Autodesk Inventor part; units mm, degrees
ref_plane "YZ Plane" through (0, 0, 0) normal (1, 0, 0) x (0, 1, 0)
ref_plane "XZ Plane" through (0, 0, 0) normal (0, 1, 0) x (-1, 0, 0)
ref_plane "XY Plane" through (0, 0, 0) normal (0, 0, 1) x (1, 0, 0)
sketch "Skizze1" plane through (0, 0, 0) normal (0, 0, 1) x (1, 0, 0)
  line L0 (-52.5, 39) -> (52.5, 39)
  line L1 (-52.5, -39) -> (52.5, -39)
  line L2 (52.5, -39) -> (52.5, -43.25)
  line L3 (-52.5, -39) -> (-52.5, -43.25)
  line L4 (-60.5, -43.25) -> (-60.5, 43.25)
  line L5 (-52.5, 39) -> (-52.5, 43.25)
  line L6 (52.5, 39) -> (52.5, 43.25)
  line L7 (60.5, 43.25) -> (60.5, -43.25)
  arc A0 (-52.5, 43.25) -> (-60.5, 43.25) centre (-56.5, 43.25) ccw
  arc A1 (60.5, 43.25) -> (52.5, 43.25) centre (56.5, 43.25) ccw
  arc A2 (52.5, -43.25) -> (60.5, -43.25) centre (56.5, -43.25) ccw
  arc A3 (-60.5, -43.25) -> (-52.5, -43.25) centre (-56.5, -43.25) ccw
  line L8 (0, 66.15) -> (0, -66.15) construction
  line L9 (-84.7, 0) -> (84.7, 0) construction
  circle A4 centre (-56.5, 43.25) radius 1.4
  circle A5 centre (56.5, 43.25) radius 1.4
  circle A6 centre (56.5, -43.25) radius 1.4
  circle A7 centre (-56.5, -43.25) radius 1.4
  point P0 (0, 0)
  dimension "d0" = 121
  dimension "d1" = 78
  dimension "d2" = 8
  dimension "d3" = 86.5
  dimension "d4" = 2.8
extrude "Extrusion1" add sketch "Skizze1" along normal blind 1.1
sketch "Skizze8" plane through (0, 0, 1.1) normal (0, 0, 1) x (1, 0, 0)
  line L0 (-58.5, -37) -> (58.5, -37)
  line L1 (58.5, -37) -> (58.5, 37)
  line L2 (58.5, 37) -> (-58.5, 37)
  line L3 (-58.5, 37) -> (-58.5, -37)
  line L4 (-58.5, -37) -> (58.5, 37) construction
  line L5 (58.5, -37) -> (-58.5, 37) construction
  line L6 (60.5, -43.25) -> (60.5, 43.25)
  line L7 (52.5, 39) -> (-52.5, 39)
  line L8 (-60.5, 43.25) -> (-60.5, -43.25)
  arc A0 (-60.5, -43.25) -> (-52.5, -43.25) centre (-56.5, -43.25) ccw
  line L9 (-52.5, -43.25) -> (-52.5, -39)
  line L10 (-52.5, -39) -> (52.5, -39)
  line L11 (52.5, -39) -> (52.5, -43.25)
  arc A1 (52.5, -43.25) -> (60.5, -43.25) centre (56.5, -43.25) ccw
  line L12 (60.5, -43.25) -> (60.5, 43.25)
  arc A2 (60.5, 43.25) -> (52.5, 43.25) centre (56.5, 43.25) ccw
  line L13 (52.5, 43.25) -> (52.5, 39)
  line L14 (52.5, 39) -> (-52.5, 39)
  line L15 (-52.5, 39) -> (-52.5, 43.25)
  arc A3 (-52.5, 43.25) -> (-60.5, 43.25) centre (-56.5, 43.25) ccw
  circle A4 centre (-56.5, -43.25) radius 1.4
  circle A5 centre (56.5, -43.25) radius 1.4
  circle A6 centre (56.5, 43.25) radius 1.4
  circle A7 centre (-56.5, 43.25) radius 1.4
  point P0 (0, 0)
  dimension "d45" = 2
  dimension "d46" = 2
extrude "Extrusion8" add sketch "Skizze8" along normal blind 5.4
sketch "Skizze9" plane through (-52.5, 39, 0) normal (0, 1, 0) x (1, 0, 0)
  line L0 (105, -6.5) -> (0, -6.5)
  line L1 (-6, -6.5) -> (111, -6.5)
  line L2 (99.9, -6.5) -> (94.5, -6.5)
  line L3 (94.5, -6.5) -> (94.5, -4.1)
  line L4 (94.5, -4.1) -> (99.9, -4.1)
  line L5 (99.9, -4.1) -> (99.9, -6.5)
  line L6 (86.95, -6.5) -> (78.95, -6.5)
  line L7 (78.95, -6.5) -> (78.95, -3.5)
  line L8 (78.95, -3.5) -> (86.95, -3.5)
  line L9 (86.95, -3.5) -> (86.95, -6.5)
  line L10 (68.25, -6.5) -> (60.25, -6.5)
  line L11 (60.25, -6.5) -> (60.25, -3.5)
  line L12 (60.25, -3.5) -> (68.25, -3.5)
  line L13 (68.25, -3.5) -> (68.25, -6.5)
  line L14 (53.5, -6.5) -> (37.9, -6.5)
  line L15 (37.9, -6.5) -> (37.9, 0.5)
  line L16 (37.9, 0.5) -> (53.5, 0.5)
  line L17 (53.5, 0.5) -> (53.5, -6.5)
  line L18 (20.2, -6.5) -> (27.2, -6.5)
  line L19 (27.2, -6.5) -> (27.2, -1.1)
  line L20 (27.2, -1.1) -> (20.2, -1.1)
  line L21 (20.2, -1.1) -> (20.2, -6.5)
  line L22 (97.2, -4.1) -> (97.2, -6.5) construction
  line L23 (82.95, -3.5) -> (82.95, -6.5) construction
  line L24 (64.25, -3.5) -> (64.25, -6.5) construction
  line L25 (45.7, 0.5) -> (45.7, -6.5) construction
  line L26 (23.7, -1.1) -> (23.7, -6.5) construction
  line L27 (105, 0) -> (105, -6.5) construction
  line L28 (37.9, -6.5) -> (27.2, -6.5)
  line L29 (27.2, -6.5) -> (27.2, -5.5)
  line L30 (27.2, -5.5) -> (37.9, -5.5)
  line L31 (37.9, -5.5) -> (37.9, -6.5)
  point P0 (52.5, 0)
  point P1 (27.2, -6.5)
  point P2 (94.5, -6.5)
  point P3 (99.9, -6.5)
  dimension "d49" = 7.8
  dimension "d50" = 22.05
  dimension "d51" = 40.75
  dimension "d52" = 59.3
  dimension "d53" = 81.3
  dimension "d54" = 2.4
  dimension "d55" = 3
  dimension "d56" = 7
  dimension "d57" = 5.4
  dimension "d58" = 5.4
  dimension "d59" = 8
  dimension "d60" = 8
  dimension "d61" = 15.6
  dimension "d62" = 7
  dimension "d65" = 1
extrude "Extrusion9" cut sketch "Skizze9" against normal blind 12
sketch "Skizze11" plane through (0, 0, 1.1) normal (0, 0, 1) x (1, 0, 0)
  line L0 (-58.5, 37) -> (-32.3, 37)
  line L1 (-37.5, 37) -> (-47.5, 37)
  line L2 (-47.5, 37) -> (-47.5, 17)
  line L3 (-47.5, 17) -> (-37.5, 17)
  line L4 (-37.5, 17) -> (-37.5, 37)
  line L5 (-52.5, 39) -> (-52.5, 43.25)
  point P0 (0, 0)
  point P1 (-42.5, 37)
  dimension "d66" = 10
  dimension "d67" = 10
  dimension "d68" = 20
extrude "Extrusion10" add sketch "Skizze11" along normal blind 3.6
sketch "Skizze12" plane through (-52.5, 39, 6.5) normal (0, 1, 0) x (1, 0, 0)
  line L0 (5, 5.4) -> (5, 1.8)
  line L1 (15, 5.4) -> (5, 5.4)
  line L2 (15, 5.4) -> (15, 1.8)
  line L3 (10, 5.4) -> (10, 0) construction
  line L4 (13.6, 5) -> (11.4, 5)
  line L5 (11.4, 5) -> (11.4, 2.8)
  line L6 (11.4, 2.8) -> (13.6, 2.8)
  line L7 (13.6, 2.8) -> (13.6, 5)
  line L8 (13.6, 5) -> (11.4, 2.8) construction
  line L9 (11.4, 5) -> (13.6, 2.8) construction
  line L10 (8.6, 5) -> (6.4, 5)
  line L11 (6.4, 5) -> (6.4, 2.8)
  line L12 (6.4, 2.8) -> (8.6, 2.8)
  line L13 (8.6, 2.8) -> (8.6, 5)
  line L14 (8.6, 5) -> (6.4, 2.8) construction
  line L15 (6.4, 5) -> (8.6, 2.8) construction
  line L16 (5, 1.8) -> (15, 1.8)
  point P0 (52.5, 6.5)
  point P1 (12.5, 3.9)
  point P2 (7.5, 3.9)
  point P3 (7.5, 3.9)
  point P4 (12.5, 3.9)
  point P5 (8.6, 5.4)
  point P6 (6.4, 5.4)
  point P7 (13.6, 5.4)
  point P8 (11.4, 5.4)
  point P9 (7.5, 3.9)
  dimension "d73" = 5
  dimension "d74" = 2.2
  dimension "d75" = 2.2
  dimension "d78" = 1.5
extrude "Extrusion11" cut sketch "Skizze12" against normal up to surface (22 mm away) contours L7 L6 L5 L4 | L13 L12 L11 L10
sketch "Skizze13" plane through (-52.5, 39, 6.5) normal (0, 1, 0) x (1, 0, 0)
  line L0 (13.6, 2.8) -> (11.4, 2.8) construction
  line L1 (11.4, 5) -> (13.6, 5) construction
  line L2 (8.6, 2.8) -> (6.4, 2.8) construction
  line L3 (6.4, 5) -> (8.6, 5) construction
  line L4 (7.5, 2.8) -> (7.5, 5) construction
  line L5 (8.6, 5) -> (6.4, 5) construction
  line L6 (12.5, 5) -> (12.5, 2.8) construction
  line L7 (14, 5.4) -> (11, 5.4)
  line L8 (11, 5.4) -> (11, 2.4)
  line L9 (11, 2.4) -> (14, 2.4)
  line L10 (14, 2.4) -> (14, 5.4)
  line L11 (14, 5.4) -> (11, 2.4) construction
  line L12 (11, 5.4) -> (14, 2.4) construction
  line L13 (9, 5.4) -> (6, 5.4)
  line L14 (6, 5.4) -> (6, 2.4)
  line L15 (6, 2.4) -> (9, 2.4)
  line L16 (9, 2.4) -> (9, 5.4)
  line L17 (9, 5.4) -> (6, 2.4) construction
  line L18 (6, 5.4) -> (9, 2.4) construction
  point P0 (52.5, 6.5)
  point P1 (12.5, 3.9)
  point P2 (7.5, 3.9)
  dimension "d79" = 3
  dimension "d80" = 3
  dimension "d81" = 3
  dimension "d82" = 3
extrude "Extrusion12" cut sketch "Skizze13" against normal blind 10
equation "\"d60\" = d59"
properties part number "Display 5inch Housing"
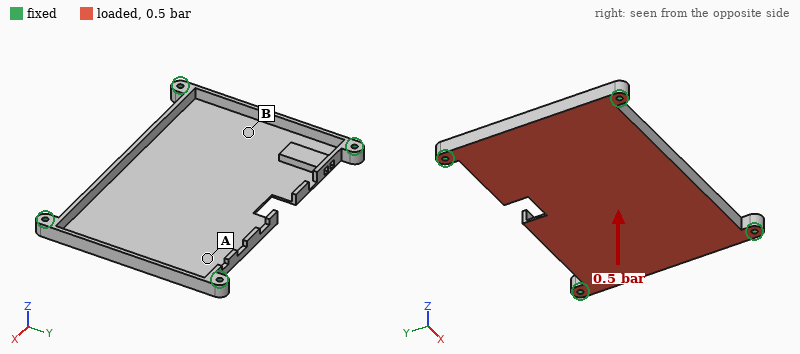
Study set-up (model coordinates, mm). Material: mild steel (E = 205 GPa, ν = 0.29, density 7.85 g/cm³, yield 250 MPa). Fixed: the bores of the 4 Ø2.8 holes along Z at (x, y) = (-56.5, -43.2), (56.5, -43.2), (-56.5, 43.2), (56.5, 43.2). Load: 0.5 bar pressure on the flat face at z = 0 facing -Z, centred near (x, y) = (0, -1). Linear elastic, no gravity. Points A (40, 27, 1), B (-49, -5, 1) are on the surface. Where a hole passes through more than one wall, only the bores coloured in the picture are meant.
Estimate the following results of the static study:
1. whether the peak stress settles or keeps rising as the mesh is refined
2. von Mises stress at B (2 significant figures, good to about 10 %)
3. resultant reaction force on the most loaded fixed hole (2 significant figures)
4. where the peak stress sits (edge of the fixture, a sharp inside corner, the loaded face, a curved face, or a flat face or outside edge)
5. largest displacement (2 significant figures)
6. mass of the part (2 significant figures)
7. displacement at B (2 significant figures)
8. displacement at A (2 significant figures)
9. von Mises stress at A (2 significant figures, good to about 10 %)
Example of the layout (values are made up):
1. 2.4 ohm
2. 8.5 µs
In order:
1. keeps rising
2. 18 MPa
3. 350 N
4. a sharp inside corner
5. 0.37 mm
6. 120 g
7. 0.070 mm
8. 0.082 mm
9. 39 MPa
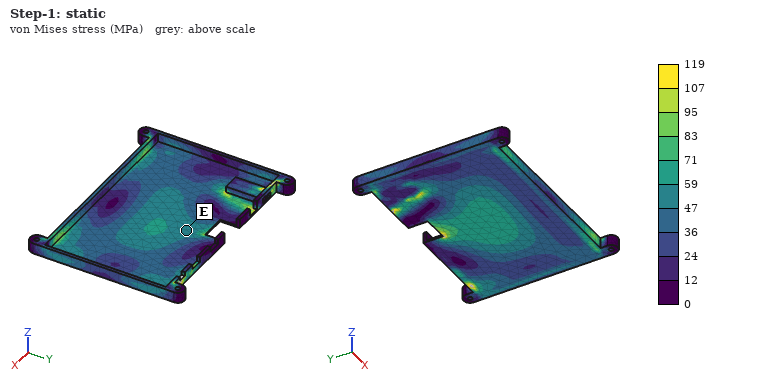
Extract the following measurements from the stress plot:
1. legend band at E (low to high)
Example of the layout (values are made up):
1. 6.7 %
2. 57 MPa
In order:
1. 47 to 59 MPa
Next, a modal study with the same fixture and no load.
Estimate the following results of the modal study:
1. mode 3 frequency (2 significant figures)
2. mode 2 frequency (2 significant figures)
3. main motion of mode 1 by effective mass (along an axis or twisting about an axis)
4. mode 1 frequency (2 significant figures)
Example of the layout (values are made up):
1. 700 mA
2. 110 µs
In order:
1. 1500 Hz
2. 1400 Hz
3. along Z
4. 780 Hz
